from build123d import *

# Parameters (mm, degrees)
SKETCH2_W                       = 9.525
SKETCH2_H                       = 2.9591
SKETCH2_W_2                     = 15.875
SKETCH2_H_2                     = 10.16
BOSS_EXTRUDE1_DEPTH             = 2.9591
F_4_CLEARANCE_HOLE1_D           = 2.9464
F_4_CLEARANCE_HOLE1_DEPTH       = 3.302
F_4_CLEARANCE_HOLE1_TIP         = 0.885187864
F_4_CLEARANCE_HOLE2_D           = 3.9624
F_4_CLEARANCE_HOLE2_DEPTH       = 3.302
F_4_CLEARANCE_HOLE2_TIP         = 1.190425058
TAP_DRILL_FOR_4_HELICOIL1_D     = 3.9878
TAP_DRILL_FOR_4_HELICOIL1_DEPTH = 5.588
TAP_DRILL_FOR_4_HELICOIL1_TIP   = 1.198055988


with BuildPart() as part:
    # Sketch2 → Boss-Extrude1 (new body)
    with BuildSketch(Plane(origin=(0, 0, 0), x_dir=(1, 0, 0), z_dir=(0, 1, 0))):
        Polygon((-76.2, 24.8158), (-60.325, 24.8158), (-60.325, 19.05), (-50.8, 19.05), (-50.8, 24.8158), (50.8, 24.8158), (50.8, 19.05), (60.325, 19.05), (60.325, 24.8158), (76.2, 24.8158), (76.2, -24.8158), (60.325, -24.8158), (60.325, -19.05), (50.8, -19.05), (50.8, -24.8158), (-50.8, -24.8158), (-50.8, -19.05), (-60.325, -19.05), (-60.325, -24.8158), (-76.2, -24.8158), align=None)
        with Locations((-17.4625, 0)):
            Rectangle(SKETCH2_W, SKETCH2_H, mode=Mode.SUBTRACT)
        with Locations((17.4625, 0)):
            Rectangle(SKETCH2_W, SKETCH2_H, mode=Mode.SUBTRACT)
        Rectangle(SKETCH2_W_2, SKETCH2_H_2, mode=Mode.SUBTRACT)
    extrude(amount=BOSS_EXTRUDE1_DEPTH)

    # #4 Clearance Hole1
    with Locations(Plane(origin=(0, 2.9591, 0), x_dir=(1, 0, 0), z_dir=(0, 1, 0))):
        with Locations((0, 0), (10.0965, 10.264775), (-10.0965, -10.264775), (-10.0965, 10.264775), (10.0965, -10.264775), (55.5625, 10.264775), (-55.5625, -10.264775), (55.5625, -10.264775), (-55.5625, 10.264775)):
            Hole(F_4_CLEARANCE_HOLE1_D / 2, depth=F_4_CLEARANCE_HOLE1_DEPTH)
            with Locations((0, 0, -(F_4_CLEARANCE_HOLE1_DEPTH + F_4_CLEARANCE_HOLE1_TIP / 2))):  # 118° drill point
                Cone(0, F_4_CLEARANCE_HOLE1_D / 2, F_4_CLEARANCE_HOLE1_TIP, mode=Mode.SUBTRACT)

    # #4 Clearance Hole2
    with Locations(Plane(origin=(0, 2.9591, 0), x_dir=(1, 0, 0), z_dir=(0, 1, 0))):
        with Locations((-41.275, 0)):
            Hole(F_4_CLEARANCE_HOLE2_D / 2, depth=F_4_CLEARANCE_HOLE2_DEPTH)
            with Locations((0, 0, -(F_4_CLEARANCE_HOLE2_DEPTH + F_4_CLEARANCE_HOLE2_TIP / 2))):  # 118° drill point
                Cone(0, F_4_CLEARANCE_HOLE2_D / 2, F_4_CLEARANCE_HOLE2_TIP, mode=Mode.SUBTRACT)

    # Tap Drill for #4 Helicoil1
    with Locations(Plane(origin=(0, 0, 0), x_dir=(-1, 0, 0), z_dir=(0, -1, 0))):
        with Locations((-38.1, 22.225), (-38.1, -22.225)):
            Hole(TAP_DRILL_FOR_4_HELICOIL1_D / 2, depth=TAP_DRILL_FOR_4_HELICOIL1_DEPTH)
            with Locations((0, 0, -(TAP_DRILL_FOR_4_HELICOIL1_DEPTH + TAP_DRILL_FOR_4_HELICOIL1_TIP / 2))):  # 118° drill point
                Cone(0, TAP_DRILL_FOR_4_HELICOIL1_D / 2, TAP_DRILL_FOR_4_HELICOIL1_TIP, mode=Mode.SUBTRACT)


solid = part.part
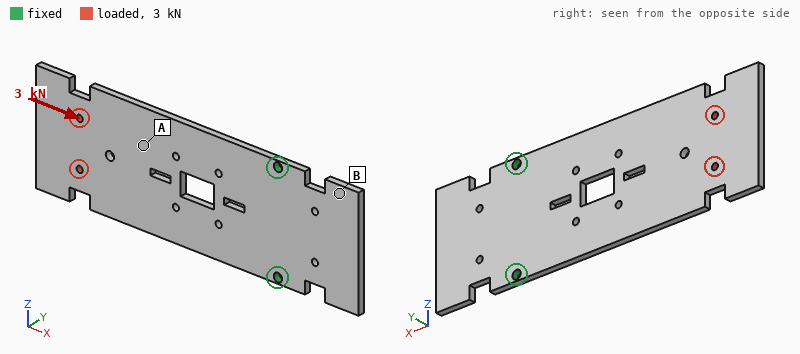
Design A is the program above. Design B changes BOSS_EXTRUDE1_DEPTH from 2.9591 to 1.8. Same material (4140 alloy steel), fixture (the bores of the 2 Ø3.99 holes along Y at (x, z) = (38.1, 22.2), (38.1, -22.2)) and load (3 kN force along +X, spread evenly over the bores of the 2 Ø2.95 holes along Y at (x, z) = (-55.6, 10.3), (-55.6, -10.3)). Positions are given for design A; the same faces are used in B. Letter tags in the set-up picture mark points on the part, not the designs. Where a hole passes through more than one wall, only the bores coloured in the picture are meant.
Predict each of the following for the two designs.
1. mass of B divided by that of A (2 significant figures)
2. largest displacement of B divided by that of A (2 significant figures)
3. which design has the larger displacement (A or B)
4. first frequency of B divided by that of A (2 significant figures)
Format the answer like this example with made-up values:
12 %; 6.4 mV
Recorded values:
0.61; 1.6; B; 0.61
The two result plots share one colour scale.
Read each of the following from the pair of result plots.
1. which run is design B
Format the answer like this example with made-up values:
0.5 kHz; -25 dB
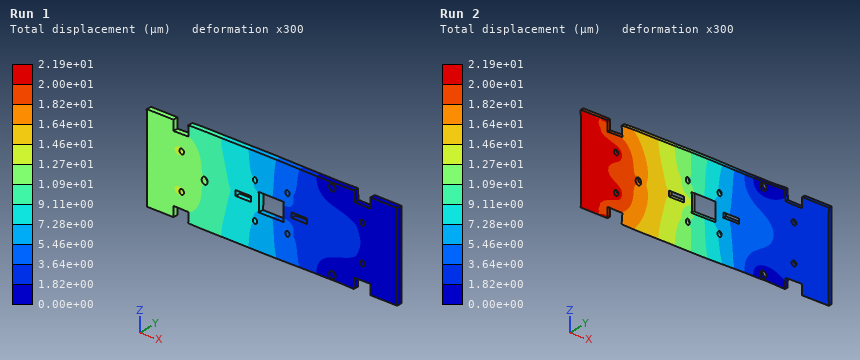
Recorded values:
Run 2
